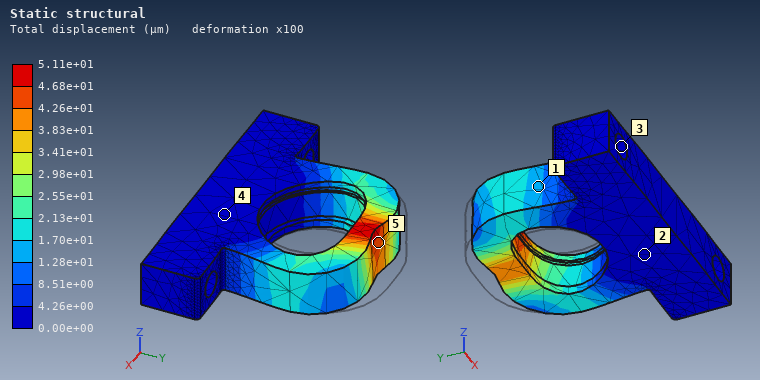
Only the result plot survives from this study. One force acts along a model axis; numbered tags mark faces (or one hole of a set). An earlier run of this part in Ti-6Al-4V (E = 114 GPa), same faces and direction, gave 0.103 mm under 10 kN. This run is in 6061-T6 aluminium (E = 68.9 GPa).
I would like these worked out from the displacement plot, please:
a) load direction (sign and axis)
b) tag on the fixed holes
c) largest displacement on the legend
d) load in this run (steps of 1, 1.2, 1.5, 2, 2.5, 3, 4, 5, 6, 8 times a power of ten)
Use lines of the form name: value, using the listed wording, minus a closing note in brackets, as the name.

load direction: -Y
tag on the fixed holes: 3
largest displacement on the legend: 5.11e+01 µm
load in this run: 3 kN
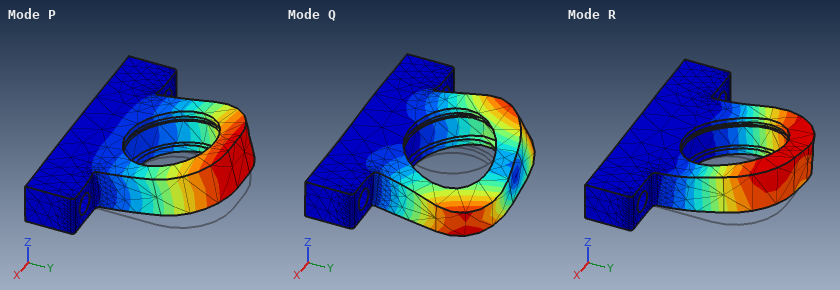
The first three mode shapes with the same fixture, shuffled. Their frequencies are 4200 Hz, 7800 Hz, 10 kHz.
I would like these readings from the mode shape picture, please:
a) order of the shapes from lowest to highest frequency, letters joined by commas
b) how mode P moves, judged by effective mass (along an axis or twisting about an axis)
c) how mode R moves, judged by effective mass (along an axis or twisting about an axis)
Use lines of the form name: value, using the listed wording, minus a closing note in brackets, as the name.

order of the shapes from lowest to highest frequency, letters joined by commas: P, R, Q
how mode P moves, judged by effective mass: along Z
how mode R moves, judged by effective mass: along X
